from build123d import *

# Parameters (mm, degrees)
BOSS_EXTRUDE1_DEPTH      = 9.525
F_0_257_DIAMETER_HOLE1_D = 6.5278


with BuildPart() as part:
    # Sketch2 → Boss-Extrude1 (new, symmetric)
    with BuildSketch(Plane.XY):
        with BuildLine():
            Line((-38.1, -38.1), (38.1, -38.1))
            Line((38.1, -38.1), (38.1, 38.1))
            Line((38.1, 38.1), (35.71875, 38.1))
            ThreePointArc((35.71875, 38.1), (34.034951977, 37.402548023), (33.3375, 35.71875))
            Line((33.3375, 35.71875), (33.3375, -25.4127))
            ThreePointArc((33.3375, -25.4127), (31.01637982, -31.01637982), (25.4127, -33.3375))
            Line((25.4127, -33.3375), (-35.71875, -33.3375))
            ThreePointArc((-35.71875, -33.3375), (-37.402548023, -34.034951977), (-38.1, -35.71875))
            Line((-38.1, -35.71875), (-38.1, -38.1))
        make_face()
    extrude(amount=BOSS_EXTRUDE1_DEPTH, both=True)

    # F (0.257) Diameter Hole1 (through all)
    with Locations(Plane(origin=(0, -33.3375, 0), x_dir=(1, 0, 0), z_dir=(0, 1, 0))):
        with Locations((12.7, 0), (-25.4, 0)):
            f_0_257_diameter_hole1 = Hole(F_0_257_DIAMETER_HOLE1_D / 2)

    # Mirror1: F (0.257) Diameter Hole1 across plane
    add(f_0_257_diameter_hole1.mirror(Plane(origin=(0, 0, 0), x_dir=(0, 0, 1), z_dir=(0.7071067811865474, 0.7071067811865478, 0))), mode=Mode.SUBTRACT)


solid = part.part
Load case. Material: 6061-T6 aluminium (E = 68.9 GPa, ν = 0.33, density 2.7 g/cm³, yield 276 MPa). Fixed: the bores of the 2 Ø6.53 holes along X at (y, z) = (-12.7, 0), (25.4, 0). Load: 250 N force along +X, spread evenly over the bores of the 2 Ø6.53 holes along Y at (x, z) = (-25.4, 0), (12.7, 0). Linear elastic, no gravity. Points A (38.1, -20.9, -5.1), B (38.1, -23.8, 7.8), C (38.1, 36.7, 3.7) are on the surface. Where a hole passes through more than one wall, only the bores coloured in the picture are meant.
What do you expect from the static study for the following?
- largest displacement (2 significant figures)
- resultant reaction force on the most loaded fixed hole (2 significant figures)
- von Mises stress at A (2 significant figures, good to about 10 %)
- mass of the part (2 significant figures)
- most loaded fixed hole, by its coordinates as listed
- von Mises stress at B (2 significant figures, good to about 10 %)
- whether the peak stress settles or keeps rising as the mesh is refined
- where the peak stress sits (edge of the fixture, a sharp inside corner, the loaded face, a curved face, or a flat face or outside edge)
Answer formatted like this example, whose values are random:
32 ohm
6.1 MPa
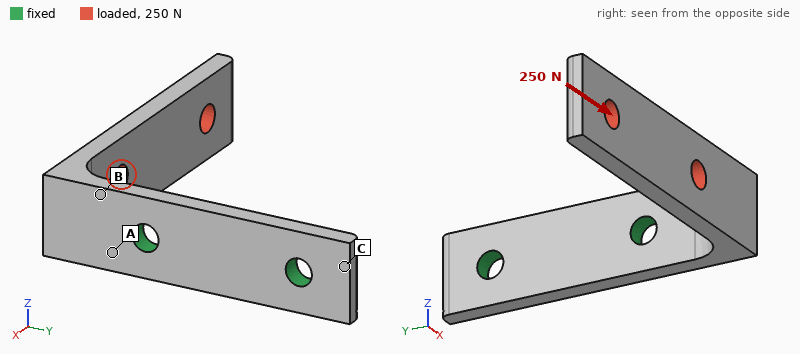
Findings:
0.34 mm
250 N
46 MPa
35 g
(-12.7, 0)
40 MPa
keeps rising
edge of the fixture
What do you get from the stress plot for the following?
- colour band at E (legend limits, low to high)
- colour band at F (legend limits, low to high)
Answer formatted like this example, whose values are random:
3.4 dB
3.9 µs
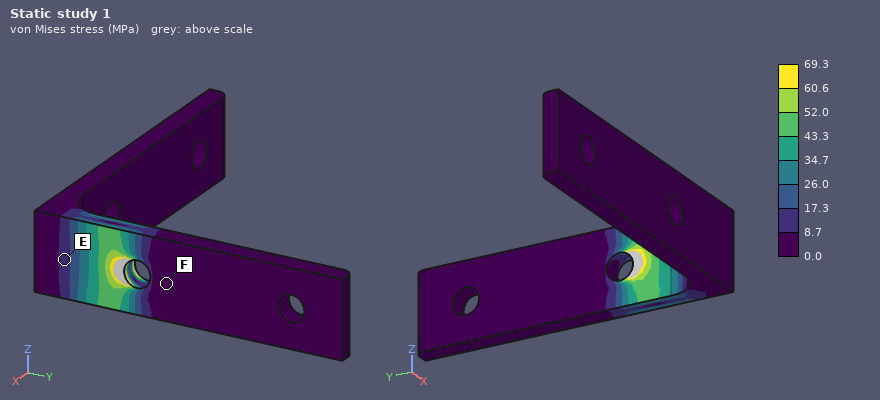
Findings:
8.7 to 17.3 MPa
0.0 to 8.7 MPa
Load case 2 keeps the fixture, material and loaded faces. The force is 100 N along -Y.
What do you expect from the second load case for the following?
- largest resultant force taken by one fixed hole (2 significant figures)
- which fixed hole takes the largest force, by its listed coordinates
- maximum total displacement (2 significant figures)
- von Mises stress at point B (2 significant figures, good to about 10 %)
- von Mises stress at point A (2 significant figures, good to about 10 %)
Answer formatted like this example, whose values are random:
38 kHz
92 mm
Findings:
95 N
(-12.7, 0)
0.83 mm
56 MPa
53 MPa
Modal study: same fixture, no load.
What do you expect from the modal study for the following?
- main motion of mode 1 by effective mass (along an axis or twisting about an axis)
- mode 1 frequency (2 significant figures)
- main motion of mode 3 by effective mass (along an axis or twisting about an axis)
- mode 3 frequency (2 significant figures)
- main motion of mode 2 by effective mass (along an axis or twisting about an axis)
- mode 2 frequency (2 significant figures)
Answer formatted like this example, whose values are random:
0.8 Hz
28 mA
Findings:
along Y
560 Hz
along X
2600 Hz
along Z
920 Hz
